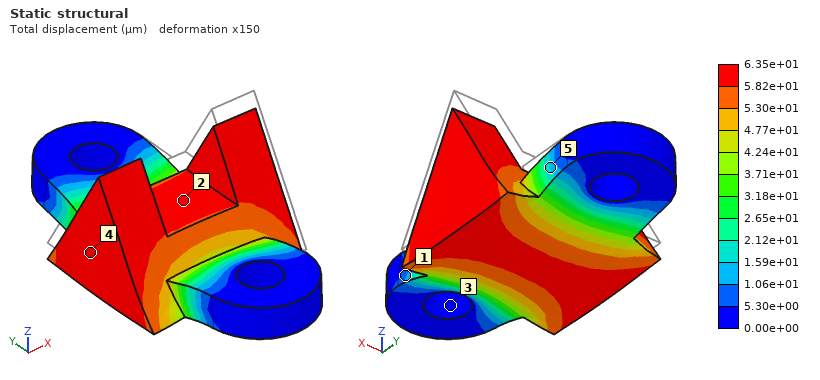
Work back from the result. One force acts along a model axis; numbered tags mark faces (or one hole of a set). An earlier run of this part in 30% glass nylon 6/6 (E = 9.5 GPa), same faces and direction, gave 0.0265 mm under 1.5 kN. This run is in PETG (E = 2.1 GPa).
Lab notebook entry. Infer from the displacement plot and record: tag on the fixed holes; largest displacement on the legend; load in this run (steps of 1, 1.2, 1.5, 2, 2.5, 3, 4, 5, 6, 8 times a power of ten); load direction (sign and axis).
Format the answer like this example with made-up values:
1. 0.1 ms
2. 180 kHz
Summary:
1. 3
2. 6.35e+01 µm
3. 800 N
4. -Z
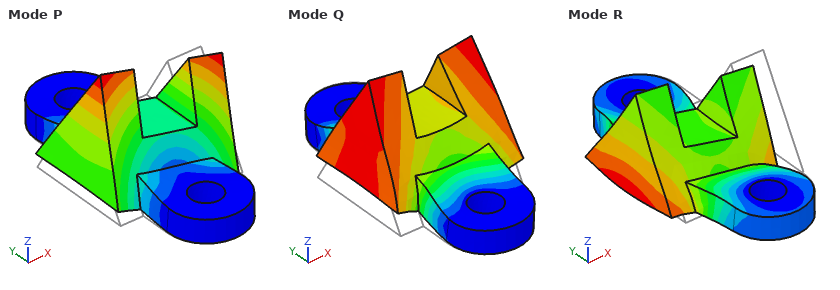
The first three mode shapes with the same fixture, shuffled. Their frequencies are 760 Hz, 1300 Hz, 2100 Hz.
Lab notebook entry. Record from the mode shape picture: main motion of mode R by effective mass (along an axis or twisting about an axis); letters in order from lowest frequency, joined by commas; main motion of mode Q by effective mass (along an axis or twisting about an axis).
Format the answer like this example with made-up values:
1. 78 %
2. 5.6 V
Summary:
1. along X
2. P, Q, R
3. along Z
